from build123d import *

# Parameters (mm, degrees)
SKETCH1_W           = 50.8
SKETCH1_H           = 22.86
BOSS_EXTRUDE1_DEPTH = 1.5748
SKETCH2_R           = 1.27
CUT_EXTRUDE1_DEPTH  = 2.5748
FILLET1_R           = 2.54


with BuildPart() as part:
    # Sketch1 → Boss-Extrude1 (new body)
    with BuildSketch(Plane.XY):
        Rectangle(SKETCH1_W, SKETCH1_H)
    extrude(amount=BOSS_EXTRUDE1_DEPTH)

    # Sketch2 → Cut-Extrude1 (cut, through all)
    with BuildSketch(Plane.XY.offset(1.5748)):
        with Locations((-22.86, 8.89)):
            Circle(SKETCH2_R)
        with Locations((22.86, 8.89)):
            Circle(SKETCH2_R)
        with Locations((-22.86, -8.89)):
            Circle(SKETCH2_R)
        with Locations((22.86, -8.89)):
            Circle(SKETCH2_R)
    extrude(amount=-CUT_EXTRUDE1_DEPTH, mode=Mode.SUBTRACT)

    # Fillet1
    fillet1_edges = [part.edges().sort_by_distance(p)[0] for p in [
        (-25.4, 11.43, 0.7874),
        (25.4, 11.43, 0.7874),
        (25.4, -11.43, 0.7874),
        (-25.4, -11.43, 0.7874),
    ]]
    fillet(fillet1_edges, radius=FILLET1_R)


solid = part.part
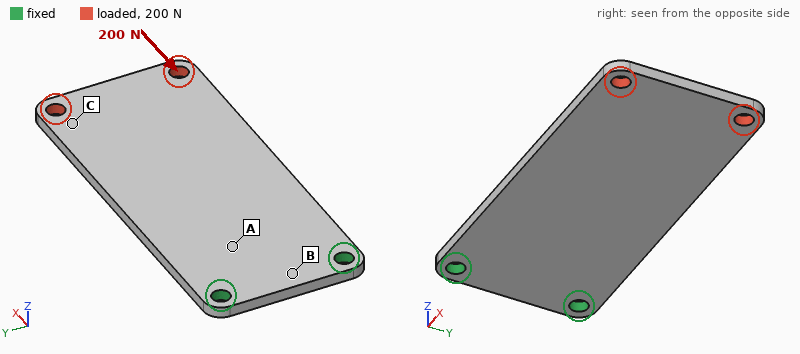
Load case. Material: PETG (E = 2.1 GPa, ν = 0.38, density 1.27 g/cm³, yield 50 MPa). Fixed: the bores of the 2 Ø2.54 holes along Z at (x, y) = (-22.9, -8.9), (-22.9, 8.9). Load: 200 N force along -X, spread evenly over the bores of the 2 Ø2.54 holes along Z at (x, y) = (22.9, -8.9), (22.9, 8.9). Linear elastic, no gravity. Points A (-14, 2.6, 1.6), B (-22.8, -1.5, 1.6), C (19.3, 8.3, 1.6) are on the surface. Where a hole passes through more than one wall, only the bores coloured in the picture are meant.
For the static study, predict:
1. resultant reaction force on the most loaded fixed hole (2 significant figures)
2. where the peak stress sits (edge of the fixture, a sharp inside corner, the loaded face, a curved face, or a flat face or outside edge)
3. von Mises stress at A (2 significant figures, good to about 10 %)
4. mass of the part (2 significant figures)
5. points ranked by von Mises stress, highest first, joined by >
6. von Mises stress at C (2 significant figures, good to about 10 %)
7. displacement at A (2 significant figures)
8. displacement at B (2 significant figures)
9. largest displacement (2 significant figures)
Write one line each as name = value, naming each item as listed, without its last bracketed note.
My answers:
resultant reaction force on the most loaded fixed hole = 100 N
where the peak stress sits = the loaded face
von Mises stress at A = 4.2 MPa
mass of the part = 2.3 g
points ranked by von Mises stress, highest first, joined by > = C > A > B
von Mises stress at C = 8.0 MPa
displacement at A = 0.038 mm
displacement at B = 0.031 mm
largest displacement = 0.18 mm
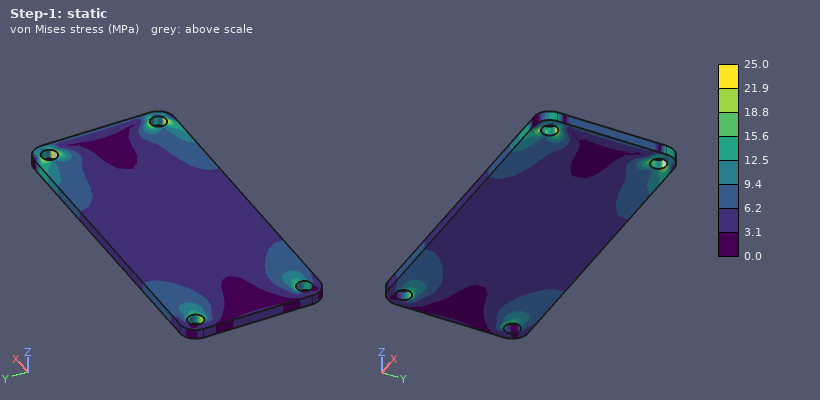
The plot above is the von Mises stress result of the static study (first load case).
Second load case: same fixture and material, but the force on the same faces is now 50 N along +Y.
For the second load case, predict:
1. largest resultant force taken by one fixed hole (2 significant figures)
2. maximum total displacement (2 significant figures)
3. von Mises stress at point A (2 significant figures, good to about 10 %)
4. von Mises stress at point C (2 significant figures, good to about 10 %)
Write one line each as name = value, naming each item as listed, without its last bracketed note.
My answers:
largest resultant force taken by one fixed hole = 130 N
maximum total displacement = 0.64 mm
von Mises stress at point A = 4.1 MPa
von Mises stress at point C = 2.6 MPa
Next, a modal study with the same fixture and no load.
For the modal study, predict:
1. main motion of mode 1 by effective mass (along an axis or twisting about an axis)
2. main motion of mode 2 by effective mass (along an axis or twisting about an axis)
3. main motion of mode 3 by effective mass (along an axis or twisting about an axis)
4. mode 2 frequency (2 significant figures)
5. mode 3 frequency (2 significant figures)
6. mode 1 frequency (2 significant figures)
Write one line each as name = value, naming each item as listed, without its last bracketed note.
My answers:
main motion of mode 1 by effective mass = along Z
main motion of mode 2 by effective mass = twisting about X
main motion of mode 3 by effective mass = along Z
mode 2 frequency = 650 Hz
mode 3 frequency = 890 Hz
mode 1 frequency = 140 Hz
